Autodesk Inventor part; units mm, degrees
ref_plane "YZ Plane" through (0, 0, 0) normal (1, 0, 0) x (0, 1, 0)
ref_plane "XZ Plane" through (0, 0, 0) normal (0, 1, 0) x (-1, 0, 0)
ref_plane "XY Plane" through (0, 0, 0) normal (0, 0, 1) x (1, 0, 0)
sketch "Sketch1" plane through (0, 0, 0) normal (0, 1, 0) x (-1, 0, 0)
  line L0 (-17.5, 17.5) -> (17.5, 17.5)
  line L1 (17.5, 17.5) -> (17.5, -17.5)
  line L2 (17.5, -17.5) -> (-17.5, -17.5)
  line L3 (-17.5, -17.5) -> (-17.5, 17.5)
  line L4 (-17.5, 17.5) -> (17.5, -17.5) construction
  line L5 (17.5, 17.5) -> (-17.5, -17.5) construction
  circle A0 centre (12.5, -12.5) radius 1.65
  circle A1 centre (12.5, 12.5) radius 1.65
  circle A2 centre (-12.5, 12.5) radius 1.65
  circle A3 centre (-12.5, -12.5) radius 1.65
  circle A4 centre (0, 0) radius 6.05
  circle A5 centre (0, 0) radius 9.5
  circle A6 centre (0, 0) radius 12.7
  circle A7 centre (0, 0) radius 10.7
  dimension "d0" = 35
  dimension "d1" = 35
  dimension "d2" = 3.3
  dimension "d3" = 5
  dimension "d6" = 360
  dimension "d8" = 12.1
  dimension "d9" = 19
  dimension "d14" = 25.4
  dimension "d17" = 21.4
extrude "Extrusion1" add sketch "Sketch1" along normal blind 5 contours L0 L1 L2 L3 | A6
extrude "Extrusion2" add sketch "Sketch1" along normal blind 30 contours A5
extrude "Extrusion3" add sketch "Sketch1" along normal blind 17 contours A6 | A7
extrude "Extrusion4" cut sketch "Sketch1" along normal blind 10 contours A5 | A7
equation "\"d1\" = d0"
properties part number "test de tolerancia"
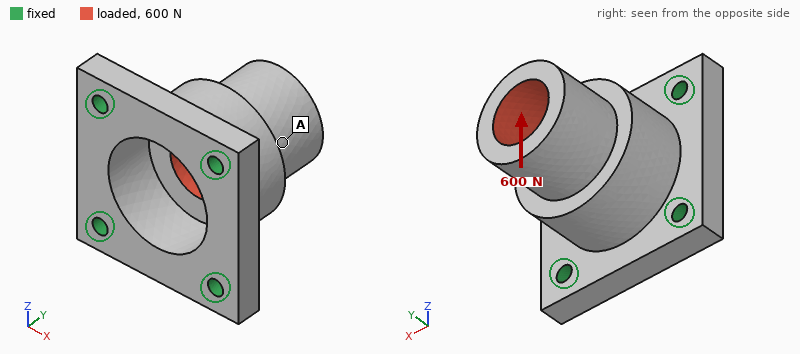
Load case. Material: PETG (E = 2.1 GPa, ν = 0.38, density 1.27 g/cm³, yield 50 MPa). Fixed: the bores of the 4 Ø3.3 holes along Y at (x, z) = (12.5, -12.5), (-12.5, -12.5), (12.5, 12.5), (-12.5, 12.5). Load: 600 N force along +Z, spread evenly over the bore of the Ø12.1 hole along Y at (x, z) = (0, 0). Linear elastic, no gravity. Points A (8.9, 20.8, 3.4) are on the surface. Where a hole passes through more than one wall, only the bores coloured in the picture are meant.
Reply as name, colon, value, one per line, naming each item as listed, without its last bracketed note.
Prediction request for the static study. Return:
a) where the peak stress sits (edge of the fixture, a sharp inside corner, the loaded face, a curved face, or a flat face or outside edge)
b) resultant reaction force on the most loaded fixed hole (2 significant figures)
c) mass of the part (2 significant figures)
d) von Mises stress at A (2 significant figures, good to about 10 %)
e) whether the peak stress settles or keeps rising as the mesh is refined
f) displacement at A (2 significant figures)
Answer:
where the peak stress sits: edge of the fixture
resultant reaction force on the most loaded fixed hole: 280 N
mass of the part: 12 g
von Mises stress at A: 4.0 MPa
whether the peak stress settles or keeps rising as the mesh is refined: keeps rising
displacement at A: 0.25 mm
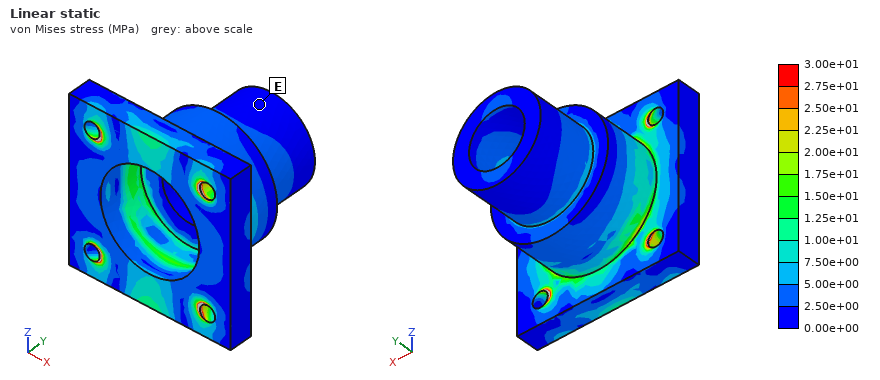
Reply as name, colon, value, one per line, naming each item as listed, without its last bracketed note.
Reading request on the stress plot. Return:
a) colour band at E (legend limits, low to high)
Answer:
colour band at E: 0.00e+00 to 2.50e+00 MPa
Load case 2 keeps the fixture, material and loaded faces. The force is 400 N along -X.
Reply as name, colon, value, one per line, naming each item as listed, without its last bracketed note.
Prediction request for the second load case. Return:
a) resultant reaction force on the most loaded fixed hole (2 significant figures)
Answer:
resultant reaction force on the most loaded fixed hole: 190 N
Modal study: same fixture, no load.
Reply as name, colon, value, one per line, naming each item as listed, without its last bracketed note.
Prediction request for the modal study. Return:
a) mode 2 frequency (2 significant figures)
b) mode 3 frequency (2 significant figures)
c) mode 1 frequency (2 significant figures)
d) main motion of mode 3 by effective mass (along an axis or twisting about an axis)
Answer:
mode 2 frequency: 3200 Hz
mode 3 frequency: 5400 Hz
mode 1 frequency: 3200 Hz
main motion of mode 3 by effective mass: along Y
